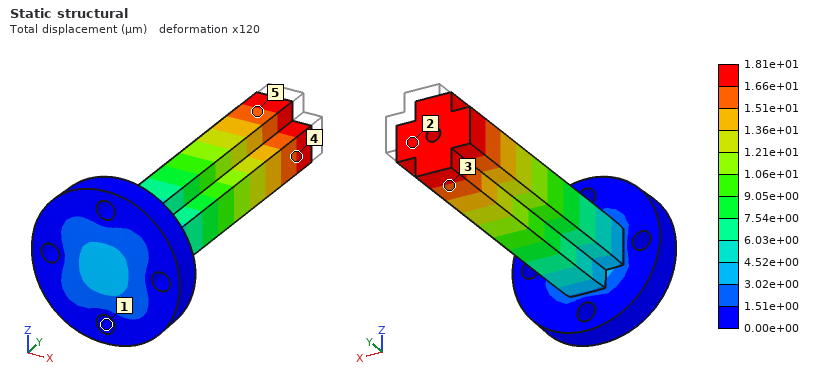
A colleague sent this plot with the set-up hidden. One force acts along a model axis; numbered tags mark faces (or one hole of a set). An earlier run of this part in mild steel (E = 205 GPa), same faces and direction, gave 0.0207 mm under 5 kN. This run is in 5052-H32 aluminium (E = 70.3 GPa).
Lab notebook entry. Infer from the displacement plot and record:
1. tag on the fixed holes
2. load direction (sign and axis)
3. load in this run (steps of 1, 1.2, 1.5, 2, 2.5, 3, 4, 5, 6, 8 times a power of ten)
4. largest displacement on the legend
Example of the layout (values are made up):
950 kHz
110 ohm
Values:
1
-Y
1.5 kN
1.81e+01 µm
